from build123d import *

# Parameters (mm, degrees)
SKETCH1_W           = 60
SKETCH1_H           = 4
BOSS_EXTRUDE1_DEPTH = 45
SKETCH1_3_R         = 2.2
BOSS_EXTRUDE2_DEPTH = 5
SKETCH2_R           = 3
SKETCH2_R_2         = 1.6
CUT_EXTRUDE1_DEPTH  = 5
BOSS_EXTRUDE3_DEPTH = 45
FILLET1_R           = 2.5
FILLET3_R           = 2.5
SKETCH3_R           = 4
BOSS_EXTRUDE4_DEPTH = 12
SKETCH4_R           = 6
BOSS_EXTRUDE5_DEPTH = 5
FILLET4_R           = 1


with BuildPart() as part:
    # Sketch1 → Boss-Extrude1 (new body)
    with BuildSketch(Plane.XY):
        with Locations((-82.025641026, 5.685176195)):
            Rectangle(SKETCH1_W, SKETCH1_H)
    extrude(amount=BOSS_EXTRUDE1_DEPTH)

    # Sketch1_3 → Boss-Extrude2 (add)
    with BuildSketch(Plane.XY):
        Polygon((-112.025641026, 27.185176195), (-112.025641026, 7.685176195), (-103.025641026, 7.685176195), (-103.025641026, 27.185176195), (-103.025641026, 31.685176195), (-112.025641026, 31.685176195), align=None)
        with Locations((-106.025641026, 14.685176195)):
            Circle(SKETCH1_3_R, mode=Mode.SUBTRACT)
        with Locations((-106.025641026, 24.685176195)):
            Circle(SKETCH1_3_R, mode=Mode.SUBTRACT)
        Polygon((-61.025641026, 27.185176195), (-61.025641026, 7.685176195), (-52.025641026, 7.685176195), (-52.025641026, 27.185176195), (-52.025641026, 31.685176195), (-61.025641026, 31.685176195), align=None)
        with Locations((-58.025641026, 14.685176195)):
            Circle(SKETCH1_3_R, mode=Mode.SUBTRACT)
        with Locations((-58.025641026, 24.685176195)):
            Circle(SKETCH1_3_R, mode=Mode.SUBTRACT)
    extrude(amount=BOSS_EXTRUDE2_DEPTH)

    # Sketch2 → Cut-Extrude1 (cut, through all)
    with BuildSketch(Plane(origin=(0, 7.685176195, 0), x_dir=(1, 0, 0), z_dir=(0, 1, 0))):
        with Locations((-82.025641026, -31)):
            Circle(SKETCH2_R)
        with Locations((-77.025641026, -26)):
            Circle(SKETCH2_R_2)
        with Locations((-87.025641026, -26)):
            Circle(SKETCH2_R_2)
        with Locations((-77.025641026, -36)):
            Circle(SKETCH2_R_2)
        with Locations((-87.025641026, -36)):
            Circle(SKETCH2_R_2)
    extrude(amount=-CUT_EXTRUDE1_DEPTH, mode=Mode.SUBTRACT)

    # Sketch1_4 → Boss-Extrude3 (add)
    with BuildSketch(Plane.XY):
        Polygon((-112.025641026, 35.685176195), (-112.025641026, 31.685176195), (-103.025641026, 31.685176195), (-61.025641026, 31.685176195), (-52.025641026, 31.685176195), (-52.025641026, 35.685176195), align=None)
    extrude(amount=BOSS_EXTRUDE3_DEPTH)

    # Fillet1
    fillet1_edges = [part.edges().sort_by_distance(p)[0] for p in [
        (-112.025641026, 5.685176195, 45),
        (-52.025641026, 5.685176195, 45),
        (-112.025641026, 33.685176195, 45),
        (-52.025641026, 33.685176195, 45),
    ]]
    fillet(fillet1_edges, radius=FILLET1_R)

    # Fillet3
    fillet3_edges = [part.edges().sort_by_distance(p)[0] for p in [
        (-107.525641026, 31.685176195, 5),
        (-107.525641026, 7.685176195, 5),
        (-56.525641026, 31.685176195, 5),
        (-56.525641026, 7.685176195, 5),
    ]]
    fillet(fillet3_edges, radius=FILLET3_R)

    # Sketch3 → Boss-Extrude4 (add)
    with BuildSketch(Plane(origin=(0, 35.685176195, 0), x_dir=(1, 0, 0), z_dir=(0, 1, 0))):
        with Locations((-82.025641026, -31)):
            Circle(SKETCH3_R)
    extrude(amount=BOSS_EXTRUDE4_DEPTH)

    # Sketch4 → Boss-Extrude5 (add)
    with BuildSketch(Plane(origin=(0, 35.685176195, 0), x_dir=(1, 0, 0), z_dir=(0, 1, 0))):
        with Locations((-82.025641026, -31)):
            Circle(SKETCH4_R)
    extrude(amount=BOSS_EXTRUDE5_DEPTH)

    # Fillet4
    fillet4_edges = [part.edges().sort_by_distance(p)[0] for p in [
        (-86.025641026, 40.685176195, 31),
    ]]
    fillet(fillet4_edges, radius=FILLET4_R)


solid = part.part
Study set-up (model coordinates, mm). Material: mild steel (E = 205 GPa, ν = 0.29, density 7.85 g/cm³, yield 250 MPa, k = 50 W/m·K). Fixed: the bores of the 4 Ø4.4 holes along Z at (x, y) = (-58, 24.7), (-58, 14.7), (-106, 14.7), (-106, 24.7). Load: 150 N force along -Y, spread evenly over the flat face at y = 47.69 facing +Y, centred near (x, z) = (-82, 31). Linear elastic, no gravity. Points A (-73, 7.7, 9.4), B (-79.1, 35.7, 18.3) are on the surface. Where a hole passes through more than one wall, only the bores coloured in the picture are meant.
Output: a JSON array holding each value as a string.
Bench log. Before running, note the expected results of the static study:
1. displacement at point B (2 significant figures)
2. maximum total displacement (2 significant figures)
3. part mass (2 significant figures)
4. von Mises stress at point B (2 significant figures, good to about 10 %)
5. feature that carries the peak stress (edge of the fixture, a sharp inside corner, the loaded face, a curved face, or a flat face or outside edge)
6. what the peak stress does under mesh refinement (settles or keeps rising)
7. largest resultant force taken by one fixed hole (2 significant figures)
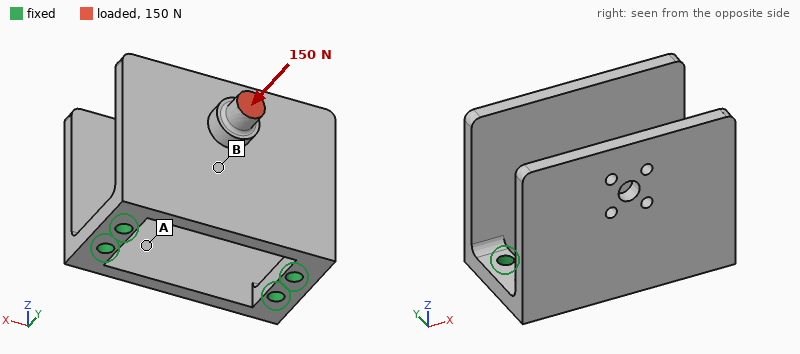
["26 µm", "76 µm", "190 g", "12 MPa", "a sharp inside corner", "keeps rising", "88 N"]
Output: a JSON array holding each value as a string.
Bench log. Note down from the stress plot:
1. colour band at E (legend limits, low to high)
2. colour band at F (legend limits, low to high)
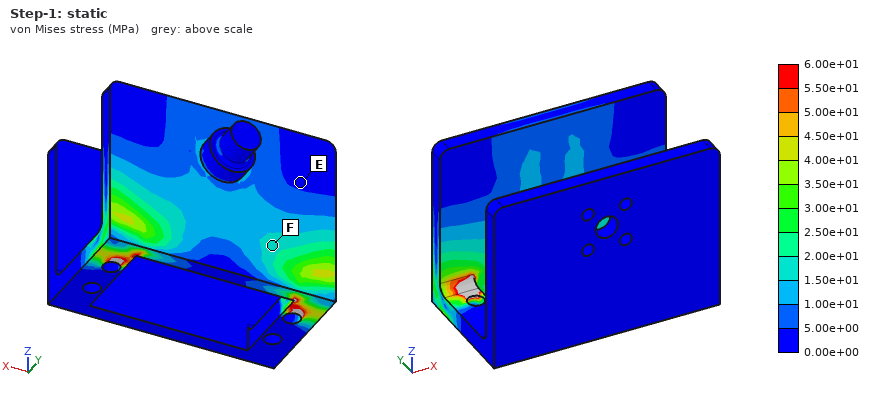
["0.00e+00 to 5.00e+00 MPa", "1.50e+01 to 2.00e+01 MPa"]
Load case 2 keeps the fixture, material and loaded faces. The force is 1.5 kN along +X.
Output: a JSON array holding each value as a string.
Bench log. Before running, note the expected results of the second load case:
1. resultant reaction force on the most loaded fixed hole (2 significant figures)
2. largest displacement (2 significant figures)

["1.3 kN", "91 µm"]
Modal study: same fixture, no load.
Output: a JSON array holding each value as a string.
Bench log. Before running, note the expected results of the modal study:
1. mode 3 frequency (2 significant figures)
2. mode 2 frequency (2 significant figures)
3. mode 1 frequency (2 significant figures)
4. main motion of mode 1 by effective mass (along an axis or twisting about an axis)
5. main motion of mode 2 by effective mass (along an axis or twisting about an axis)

["3100 Hz", "1200 Hz", "1100 Hz", "along Y", "along Y"]
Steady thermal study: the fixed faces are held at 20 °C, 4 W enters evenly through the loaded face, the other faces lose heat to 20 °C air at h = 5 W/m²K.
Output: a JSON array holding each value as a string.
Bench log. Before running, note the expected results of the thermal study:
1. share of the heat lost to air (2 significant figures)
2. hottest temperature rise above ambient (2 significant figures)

["11 %", "35 K"]
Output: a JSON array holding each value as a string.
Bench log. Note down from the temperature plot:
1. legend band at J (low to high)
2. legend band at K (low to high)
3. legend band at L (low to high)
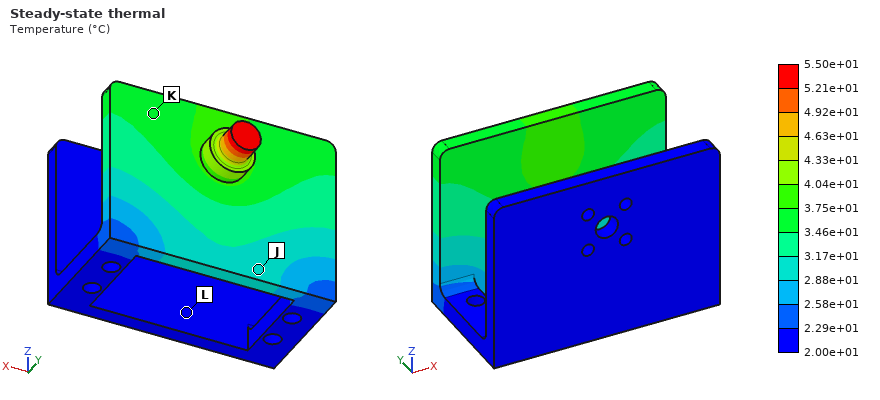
["2.88e+01 to 3.17e+01 °C", "3.46e+01 to 3.75e+01 °C", "2.00e+01 to 2.29e+01 °C"]
